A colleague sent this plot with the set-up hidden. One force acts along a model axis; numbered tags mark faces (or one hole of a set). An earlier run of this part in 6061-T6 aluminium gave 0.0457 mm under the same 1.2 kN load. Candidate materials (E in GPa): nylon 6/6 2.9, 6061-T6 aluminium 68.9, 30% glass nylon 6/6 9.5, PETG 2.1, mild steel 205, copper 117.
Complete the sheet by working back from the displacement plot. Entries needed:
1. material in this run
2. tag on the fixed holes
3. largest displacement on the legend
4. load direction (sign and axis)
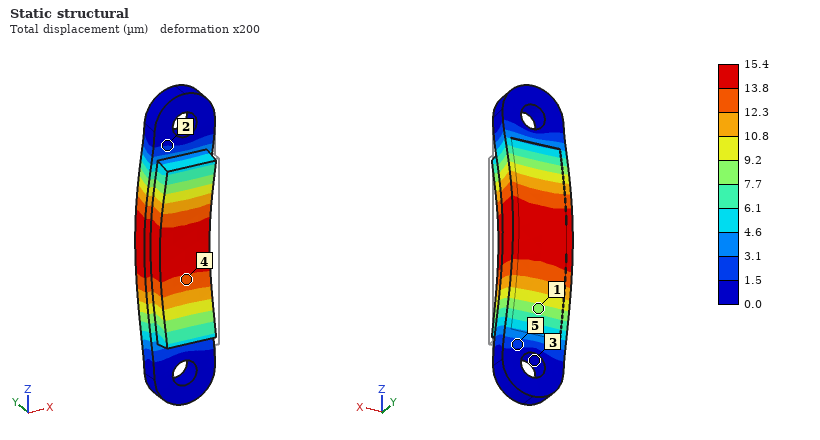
mild steel
3
15.4 µm
+Y
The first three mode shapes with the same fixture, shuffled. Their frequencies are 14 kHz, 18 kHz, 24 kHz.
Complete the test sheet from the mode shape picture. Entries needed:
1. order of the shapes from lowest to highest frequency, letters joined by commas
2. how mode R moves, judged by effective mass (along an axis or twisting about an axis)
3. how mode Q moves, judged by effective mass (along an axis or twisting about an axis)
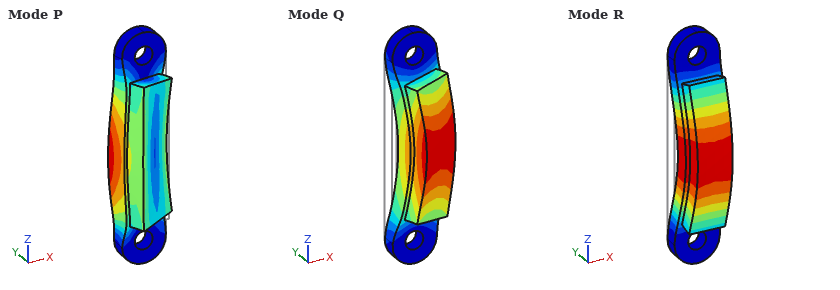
R, Q, P
along Y
along X
